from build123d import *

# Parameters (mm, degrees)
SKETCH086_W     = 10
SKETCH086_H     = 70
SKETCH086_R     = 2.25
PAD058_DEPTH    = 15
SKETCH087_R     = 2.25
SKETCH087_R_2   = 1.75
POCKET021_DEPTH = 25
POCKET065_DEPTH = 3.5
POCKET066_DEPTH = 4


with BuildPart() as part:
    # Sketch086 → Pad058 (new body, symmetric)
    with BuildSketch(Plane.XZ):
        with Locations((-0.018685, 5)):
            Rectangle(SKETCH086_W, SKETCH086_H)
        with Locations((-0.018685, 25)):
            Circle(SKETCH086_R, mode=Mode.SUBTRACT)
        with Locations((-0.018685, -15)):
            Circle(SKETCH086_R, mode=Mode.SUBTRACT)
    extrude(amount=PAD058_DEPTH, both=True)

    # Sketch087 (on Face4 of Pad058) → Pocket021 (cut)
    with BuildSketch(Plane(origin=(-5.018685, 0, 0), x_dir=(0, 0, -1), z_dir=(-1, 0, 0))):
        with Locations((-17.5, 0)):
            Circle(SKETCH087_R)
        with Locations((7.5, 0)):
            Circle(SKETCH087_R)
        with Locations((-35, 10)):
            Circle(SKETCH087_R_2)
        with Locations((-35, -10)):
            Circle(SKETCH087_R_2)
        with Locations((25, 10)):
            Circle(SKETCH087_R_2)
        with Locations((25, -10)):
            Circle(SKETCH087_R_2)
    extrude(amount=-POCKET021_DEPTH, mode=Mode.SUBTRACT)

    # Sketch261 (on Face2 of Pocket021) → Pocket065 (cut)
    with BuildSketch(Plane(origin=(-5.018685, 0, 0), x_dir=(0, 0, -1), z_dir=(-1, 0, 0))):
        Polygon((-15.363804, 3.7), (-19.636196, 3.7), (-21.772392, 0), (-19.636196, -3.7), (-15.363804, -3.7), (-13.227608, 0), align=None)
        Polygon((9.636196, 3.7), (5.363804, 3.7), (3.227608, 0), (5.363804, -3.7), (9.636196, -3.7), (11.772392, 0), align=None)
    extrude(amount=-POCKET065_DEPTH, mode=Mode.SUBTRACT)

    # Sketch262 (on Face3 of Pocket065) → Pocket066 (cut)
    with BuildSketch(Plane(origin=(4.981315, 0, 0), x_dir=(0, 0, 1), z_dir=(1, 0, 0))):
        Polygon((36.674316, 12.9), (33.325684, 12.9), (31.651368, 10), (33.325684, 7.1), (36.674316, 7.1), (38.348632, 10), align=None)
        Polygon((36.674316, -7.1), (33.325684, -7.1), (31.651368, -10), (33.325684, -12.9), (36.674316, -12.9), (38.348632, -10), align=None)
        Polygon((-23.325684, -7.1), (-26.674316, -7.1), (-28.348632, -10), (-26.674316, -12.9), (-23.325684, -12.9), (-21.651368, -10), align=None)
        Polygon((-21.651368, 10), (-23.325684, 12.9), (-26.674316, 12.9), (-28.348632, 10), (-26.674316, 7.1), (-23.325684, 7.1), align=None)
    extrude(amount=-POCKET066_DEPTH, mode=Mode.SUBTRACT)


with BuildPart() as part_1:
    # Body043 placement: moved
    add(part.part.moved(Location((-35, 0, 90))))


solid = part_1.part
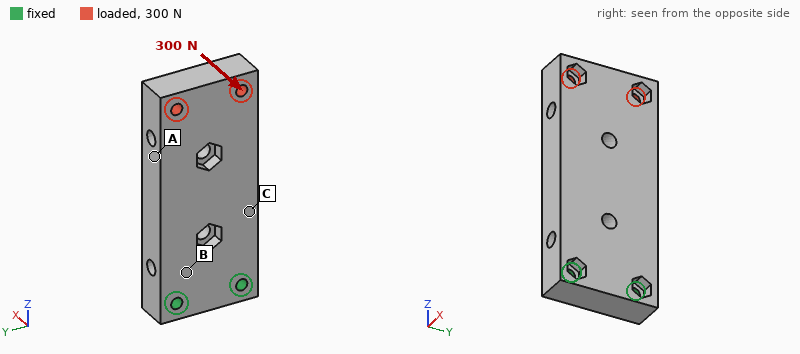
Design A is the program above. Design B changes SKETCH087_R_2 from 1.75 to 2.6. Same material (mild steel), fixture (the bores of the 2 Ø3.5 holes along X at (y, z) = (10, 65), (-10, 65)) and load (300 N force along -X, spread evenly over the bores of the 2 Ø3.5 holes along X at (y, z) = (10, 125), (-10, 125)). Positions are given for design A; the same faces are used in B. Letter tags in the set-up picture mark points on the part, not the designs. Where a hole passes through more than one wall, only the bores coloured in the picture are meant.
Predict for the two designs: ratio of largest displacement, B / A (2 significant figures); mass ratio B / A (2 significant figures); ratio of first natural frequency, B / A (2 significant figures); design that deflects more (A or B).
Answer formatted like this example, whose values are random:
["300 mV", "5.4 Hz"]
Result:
["0.85", "0.99", "1.1", "A"]
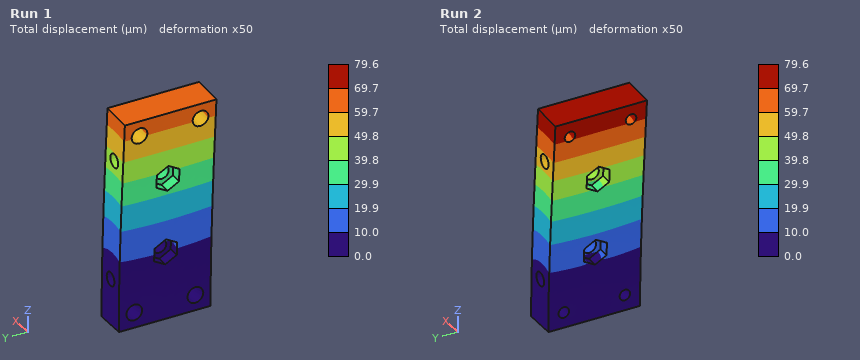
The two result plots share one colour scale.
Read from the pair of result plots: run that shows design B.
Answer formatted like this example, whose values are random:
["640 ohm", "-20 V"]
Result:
["Run 1"]
